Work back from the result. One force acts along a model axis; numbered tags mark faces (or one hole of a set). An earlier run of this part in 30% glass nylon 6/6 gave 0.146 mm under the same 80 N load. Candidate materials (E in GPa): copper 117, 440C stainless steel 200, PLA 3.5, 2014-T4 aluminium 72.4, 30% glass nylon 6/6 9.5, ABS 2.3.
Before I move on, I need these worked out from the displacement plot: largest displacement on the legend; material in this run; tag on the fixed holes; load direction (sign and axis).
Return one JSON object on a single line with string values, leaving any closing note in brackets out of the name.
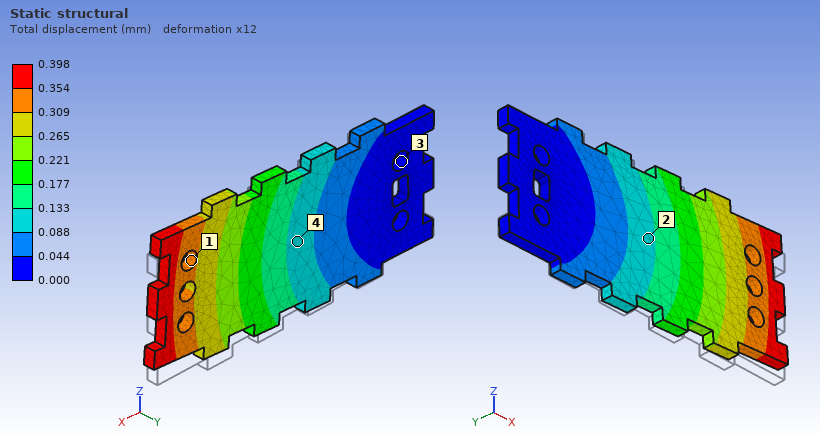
{"largest displacement on the legend": "0.398 mm", "material in this run": "PLA", "tag on the fixed holes": "3", "load direction": "+Z"}
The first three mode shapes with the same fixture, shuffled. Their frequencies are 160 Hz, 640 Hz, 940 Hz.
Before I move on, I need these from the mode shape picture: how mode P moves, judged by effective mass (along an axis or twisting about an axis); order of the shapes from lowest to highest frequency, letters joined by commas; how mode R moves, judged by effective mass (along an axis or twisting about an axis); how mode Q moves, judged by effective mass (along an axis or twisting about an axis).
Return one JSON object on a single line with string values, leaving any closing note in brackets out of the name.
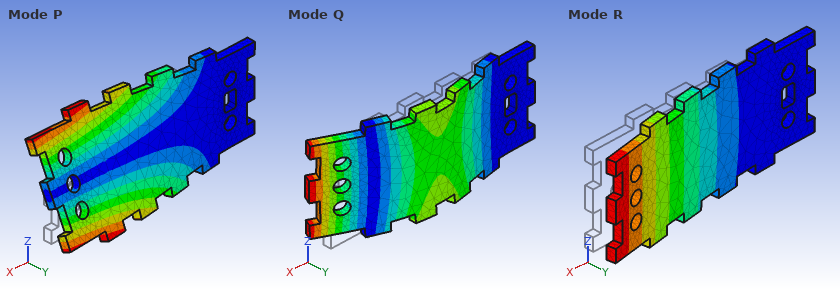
{"how mode P moves, judged by effective mass": "twisting about X", "order of the shapes from lowest to highest frequency, letters joined by commas": "R, P, Q", "how mode R moves, judged by effective mass": "along Y", "how mode Q moves, judged by effective mass": "along Y"}
